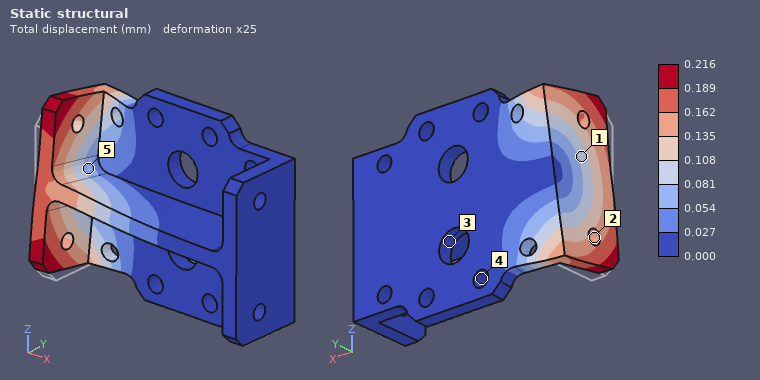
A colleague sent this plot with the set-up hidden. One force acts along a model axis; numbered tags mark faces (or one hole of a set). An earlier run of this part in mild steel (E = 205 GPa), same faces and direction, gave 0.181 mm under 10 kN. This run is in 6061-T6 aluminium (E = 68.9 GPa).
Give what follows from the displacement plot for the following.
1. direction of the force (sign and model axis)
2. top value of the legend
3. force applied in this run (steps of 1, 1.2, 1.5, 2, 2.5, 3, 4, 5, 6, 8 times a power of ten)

+Z
0.216 mm
4 kN
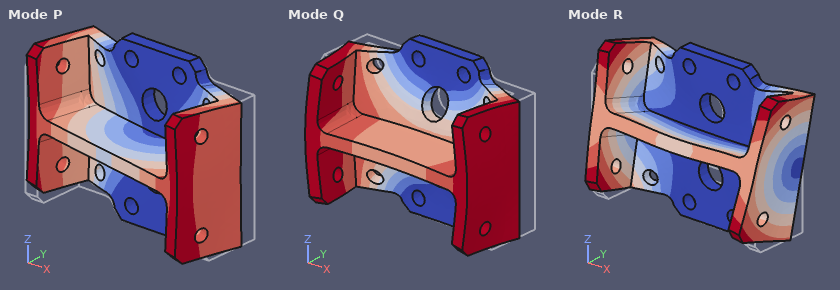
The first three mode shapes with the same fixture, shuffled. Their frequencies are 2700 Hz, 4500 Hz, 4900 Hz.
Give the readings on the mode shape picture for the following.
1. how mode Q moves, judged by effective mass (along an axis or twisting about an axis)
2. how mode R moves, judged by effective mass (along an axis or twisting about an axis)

along Y
along Z
